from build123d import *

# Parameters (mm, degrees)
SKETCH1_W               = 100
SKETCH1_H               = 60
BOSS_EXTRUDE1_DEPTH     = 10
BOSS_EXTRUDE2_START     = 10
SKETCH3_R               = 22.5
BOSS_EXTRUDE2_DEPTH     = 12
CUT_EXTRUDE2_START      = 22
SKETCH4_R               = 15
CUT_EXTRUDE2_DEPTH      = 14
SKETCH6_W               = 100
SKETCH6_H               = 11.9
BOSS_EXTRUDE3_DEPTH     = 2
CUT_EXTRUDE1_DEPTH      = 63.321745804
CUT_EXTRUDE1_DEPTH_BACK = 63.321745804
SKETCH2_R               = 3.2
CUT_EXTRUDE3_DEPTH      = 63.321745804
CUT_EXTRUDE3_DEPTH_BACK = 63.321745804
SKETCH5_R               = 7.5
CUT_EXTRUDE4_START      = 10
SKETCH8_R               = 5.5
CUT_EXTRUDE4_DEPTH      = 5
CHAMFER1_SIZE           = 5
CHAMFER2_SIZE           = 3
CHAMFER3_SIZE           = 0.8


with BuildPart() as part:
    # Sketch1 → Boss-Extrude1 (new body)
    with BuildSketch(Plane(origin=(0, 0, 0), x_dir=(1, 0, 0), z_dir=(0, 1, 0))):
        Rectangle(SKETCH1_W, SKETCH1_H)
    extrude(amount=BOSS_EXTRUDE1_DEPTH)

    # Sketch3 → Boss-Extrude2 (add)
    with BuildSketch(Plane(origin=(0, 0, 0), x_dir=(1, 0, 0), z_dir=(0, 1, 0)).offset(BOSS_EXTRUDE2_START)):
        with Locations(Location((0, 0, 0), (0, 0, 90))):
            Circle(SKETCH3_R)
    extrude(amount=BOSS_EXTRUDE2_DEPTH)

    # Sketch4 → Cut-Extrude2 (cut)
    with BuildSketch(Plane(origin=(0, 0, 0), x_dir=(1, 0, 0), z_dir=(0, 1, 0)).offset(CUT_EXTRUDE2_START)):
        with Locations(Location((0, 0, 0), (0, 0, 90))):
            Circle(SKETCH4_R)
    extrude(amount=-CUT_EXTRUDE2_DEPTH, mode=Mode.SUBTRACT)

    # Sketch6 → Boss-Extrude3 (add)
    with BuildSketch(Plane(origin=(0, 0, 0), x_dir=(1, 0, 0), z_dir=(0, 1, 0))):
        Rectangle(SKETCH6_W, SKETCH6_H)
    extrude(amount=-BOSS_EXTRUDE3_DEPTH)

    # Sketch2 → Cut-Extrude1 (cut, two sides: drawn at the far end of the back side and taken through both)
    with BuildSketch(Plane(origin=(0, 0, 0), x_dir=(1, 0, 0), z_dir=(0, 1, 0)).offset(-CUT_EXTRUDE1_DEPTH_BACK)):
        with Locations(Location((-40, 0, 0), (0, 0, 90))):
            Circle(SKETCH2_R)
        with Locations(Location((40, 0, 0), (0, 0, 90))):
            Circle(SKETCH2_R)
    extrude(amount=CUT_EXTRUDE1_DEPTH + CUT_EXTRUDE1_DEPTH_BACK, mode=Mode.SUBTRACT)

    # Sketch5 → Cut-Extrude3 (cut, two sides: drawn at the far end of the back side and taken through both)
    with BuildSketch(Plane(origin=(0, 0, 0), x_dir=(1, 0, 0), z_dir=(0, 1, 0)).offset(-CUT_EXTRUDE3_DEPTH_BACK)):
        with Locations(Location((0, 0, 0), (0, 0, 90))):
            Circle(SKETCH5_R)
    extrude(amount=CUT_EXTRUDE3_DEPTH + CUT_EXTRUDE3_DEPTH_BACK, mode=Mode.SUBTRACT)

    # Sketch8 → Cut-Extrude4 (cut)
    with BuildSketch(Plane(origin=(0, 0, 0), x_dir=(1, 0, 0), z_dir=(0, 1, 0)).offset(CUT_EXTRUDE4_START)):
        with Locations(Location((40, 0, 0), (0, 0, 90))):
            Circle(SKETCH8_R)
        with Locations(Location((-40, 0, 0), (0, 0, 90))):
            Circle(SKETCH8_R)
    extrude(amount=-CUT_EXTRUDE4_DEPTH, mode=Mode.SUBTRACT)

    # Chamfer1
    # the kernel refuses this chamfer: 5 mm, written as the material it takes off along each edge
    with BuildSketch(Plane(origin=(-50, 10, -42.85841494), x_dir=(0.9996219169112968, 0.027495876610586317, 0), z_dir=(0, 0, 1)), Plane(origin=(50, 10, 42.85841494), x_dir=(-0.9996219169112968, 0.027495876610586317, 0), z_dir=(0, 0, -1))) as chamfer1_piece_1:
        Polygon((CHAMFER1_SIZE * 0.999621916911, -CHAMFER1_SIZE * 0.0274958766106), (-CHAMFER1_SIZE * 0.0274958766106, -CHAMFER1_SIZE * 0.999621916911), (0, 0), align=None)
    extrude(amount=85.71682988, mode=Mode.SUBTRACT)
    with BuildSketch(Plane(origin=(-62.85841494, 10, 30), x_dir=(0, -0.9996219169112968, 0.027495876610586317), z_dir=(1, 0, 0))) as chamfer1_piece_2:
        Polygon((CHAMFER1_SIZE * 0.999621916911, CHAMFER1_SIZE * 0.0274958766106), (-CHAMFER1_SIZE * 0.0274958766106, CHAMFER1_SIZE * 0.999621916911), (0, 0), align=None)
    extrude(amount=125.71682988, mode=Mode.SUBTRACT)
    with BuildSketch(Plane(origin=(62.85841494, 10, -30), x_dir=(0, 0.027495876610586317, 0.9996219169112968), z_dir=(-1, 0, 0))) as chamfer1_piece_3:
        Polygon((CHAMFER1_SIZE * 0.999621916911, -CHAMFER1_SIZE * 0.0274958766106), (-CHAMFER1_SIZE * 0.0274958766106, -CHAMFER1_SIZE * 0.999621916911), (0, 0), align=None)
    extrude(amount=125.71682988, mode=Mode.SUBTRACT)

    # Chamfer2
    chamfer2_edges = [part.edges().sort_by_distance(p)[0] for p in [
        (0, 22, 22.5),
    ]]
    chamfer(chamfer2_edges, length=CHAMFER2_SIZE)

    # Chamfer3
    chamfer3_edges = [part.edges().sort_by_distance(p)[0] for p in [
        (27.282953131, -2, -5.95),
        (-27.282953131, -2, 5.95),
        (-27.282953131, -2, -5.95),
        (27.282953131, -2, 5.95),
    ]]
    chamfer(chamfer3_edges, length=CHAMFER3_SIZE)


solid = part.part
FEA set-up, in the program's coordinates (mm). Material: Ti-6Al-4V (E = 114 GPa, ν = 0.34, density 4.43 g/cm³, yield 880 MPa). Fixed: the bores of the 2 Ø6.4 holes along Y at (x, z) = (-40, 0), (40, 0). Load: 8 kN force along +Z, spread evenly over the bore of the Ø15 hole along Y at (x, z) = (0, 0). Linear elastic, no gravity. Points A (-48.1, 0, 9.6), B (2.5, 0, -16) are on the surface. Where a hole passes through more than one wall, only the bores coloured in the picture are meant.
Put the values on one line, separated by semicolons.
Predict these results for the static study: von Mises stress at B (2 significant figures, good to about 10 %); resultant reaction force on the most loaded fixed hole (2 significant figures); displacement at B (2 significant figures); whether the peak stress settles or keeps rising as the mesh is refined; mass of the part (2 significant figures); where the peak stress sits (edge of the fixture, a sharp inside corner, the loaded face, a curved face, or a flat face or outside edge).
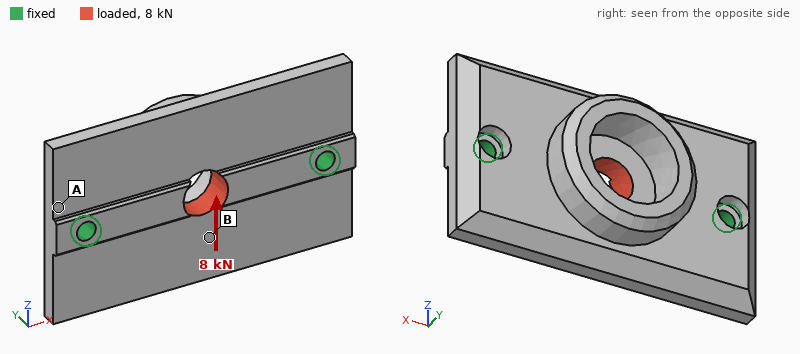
17 MPa; 4.0 kN; 12 µm; keeps rising; 280 g; edge of the fixture
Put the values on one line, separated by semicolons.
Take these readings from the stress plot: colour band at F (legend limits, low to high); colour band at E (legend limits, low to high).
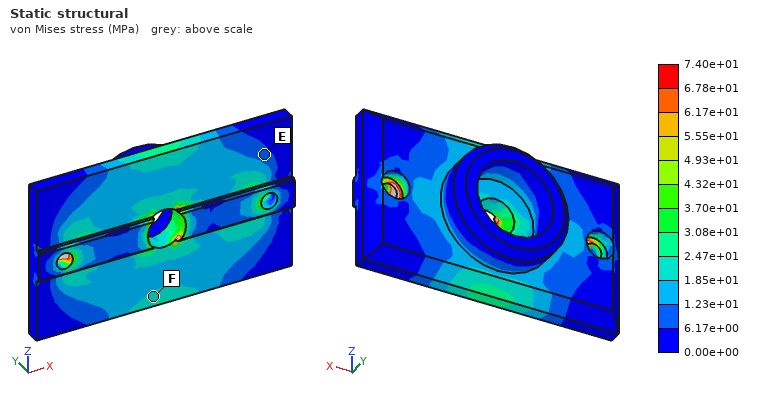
1.85e+01 to 2.47e+01 MPa; 6.17e+00 to 1.23e+01 MPa
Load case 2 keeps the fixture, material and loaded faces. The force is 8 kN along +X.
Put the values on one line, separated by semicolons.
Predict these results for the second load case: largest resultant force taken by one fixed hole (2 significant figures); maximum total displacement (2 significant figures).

4.0 kN; 6.9 µm
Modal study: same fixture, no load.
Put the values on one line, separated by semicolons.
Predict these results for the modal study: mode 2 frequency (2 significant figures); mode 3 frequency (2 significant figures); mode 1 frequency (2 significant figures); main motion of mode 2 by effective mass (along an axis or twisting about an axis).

5400 Hz; 8400 Hz; 3300 Hz; along Y
